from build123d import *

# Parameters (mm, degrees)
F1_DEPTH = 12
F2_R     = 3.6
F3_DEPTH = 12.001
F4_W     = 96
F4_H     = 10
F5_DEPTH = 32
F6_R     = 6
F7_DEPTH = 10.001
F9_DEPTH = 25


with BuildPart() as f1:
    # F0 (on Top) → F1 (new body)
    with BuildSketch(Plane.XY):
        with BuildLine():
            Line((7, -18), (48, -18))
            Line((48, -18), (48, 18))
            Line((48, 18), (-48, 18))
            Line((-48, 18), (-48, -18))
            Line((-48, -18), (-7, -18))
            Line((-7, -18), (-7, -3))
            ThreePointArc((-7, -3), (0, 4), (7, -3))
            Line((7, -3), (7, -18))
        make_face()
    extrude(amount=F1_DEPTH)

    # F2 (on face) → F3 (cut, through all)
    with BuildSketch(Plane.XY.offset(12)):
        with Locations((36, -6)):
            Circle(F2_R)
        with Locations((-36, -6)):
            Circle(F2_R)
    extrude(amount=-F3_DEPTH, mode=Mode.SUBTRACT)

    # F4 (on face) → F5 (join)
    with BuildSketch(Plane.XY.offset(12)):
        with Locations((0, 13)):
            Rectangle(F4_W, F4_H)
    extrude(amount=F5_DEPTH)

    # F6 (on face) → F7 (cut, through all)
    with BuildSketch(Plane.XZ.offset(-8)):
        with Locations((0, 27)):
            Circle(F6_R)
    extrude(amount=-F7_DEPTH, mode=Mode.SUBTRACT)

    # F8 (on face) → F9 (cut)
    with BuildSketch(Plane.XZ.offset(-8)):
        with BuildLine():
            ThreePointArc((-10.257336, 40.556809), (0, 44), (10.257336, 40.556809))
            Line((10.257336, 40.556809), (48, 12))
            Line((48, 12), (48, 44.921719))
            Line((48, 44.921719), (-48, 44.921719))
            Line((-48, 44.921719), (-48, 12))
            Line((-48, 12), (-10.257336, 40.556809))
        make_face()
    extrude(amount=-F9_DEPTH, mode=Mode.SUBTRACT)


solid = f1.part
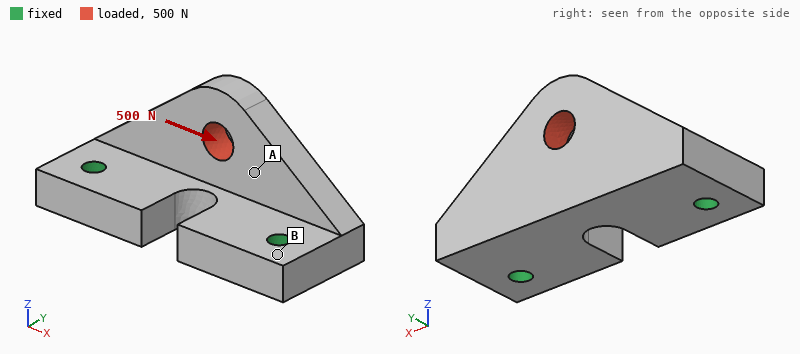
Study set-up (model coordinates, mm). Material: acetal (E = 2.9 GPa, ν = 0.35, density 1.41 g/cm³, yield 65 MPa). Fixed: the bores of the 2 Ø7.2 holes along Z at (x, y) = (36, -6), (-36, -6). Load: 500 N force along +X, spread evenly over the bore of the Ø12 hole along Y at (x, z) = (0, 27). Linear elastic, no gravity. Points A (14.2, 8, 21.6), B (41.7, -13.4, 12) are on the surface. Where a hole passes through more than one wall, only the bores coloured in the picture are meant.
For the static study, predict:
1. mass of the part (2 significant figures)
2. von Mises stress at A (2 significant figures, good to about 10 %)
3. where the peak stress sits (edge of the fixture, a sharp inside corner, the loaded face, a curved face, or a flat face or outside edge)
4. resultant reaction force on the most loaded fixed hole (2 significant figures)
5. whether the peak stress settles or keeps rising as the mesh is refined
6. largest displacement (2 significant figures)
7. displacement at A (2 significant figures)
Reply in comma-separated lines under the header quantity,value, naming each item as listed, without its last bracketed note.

quantity,value
mass of the part,75 g
von Mises stress at A,1.8 MPa
where the peak stress sits,edge of the fixture
resultant reaction force on the most loaded fixed hole,310 N
whether the peak stress settles or keeps rising as the mesh is refined,keeps rising
largest displacement,60 µm
displacement at A,36 µm
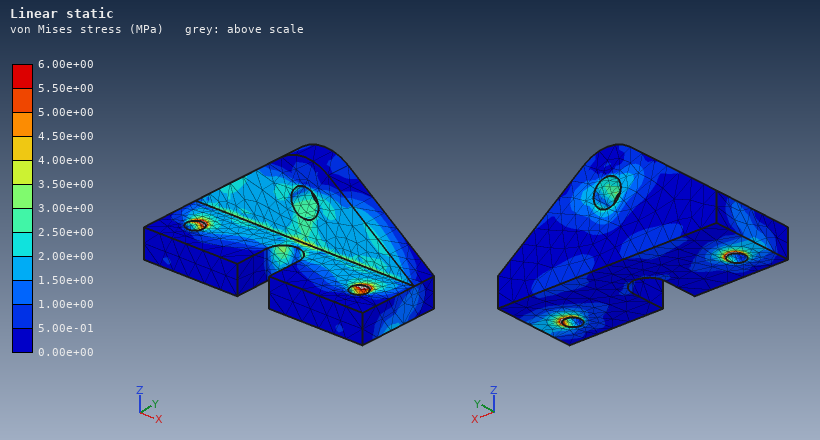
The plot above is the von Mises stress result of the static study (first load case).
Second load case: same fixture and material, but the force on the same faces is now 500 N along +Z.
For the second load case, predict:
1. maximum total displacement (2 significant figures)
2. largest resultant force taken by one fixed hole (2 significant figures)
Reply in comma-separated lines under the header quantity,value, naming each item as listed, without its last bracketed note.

quantity,value
maximum total displacement,0.20 mm
largest resultant force taken by one fixed hole,250 N
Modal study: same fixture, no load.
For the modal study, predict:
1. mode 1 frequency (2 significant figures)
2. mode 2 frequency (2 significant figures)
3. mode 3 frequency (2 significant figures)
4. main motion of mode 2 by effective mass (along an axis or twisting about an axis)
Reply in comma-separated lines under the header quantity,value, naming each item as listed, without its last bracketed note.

quantity,value
mode 1 frequency,1400 Hz
mode 2 frequency,2600 Hz
mode 3 frequency,2800 Hz
main motion of mode 2 by effective mass,along Z
